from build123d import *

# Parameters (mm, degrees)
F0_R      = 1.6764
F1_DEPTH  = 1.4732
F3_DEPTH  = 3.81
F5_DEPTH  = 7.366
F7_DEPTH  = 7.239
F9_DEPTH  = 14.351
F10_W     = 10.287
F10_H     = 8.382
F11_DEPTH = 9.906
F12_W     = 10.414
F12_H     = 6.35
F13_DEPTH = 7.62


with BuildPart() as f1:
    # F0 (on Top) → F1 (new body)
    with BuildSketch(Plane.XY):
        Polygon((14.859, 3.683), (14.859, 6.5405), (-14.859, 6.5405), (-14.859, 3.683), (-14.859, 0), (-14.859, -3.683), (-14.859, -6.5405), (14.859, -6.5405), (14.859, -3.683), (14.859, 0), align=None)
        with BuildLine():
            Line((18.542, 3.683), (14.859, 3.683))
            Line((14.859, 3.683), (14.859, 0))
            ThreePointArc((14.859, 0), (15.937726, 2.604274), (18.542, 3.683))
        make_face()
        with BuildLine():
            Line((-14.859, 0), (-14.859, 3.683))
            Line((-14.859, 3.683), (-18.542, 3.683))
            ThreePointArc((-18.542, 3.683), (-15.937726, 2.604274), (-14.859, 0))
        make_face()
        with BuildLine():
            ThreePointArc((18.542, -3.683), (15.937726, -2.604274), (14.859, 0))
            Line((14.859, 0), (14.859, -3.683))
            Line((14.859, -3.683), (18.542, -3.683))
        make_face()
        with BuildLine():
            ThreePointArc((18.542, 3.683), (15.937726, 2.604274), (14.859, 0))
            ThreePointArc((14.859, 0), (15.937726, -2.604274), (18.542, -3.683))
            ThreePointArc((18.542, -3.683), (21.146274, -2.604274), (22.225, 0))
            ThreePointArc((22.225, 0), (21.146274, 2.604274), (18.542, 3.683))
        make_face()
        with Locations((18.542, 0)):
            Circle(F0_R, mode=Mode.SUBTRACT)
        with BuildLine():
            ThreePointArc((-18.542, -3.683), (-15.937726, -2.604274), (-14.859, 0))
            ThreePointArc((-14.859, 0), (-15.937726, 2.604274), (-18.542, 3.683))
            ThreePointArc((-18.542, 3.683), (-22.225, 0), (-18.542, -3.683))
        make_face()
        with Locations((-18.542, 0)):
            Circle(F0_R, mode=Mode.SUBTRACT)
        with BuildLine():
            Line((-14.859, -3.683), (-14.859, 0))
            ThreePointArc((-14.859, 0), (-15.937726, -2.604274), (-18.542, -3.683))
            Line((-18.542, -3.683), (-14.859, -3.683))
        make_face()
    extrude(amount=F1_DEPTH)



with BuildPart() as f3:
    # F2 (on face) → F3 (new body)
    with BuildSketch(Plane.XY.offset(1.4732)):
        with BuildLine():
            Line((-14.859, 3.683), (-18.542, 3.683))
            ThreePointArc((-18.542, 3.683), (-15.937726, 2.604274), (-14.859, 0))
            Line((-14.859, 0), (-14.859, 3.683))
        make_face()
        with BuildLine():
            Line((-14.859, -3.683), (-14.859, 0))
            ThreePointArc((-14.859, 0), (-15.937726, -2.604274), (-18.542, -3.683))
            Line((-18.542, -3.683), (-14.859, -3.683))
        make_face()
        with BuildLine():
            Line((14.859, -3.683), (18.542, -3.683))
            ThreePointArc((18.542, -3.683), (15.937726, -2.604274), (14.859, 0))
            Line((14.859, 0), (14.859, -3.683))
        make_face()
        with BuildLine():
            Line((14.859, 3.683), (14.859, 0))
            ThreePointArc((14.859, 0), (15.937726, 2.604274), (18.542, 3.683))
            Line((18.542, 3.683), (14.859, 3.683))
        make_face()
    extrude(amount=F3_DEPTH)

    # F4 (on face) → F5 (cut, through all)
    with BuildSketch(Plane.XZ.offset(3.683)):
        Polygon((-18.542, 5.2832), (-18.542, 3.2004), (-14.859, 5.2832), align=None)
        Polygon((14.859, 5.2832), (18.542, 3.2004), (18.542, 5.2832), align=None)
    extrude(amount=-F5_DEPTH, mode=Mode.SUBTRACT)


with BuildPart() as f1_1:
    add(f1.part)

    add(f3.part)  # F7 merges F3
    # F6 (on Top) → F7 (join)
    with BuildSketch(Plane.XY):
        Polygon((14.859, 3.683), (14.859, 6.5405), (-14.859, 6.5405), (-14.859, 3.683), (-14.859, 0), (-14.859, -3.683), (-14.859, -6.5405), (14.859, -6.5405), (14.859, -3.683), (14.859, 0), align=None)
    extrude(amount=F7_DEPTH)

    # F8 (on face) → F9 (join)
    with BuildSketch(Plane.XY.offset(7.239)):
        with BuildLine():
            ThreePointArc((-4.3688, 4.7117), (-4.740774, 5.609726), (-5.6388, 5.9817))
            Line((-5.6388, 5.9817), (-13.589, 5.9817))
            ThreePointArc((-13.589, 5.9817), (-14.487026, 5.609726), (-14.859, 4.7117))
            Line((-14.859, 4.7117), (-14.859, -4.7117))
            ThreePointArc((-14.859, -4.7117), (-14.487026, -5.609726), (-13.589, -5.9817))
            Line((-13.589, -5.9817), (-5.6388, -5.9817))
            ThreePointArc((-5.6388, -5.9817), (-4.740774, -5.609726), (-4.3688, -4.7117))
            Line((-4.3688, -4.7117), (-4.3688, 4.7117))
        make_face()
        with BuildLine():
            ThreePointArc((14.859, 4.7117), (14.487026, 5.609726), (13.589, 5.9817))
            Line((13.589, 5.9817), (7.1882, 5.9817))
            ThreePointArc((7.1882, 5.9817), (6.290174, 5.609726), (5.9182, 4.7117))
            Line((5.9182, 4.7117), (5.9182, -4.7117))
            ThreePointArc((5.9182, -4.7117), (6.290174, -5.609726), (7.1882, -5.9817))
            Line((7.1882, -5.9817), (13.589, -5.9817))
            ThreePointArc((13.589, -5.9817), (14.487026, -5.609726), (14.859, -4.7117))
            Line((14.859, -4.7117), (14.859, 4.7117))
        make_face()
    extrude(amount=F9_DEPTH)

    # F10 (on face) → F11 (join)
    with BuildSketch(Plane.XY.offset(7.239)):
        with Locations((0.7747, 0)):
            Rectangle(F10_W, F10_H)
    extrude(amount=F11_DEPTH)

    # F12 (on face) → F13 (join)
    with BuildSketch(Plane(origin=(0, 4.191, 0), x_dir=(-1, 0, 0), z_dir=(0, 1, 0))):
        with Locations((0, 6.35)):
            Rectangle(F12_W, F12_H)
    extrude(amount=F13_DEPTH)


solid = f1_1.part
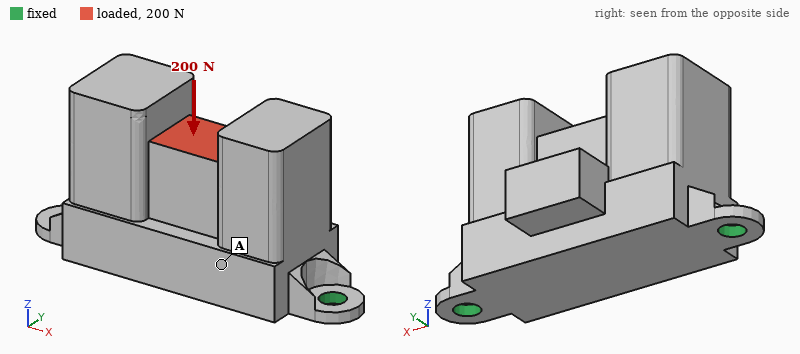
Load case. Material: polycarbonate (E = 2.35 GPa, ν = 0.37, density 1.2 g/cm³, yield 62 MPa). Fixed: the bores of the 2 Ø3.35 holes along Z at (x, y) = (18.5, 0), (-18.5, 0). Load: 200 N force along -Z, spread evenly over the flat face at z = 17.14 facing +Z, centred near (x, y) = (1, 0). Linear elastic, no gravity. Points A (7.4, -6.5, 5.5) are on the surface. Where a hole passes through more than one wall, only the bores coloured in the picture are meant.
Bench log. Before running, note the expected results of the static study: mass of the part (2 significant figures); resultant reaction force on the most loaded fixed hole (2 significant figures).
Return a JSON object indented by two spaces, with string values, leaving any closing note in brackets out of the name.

{
  "mass of the part": "9.0 g",
  "resultant reaction force on the most loaded fixed hole": "120 N"
}
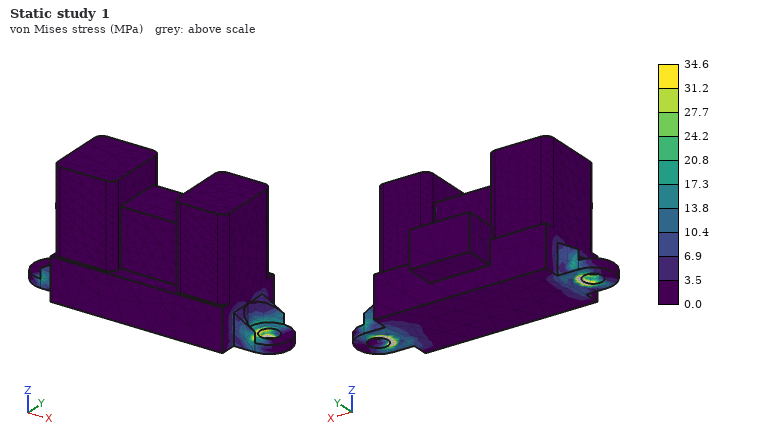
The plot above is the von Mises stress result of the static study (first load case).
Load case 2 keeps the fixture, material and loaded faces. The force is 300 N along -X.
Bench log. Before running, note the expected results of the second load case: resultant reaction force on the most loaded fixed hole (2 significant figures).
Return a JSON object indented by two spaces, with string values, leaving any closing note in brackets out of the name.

{
  "resultant reaction force on the most loaded fixed hole": "210 N"
}
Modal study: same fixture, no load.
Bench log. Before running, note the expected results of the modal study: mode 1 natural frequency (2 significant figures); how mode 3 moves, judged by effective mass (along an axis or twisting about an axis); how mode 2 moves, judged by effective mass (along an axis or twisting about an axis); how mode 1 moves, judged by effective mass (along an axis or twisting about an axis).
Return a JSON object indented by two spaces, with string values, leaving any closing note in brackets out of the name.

{
  "mode 1 natural frequency": "570 Hz",
  "how mode 3 moves, judged by effective mass": "along X",
  "how mode 2 moves, judged by effective mass": "along Z",
  "how mode 1 moves, judged by effective mass": "along Y"
}
